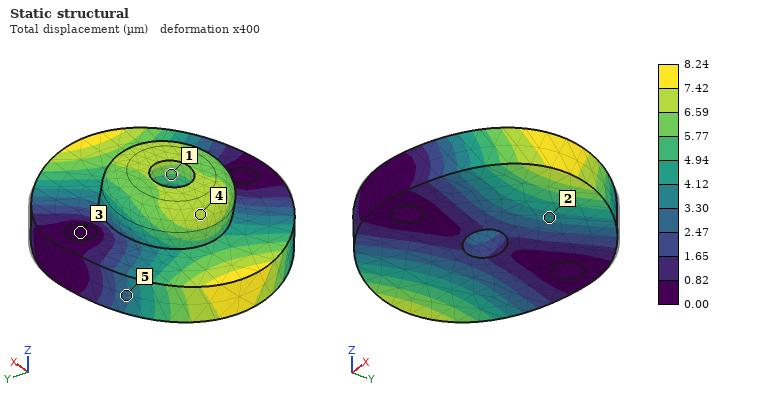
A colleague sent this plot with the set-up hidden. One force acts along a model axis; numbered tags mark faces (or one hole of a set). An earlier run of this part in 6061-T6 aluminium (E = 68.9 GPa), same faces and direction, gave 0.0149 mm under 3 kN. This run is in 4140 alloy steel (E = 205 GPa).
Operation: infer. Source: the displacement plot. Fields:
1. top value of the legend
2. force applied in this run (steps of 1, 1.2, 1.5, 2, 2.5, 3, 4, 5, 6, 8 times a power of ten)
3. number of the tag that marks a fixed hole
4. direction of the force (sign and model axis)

8.24 µm
5 kN
3
-X
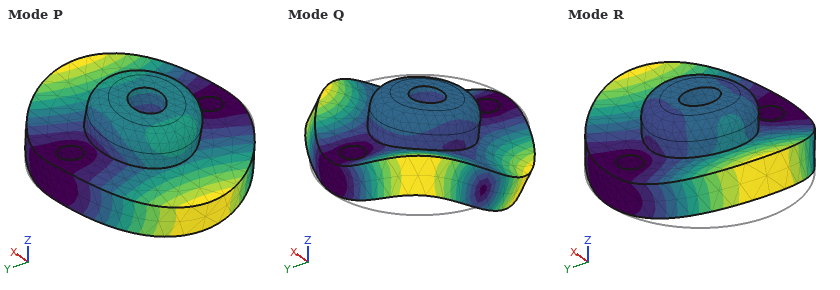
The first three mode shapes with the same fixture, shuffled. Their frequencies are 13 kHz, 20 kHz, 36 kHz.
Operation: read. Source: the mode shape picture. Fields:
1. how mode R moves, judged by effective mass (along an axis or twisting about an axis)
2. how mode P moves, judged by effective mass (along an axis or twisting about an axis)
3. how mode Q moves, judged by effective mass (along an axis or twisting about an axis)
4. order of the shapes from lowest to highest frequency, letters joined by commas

along Z
twisting about Y
twisting about X
P, R, Q
